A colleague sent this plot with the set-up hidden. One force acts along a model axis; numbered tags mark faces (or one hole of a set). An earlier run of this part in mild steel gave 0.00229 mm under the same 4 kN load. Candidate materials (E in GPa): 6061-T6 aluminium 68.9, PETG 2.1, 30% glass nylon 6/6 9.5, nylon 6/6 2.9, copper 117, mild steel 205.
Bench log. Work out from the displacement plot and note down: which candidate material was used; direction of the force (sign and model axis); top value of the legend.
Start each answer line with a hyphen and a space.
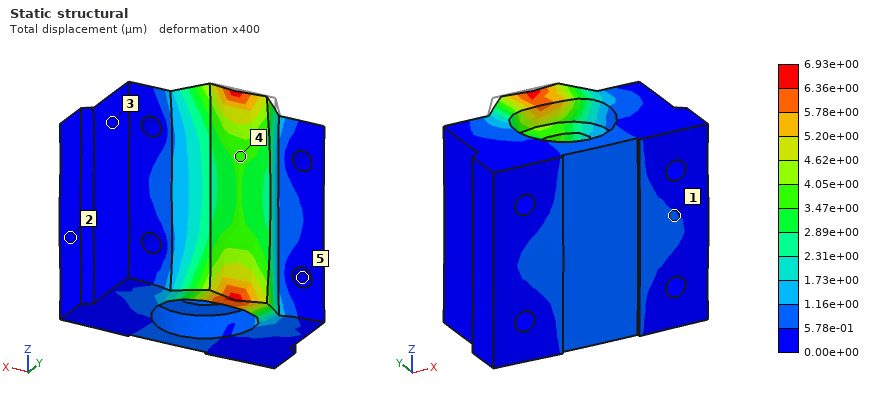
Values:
- 6061-T6 aluminium
- -Y
- 6.93e+00 µm
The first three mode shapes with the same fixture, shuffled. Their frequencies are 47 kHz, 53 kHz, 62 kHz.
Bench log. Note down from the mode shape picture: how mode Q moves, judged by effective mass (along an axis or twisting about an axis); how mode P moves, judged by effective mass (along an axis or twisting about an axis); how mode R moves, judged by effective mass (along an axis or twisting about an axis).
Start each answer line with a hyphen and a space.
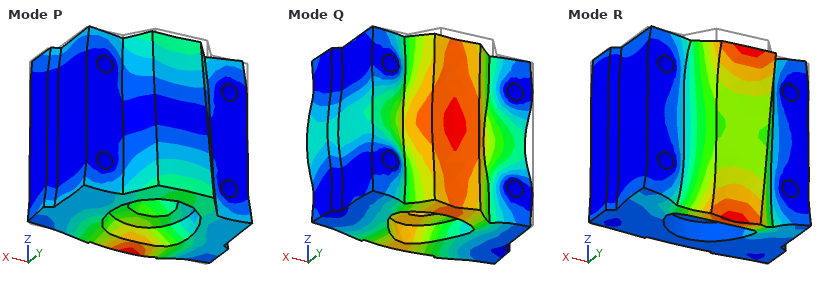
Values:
- along Y
- along Z
- along Z
